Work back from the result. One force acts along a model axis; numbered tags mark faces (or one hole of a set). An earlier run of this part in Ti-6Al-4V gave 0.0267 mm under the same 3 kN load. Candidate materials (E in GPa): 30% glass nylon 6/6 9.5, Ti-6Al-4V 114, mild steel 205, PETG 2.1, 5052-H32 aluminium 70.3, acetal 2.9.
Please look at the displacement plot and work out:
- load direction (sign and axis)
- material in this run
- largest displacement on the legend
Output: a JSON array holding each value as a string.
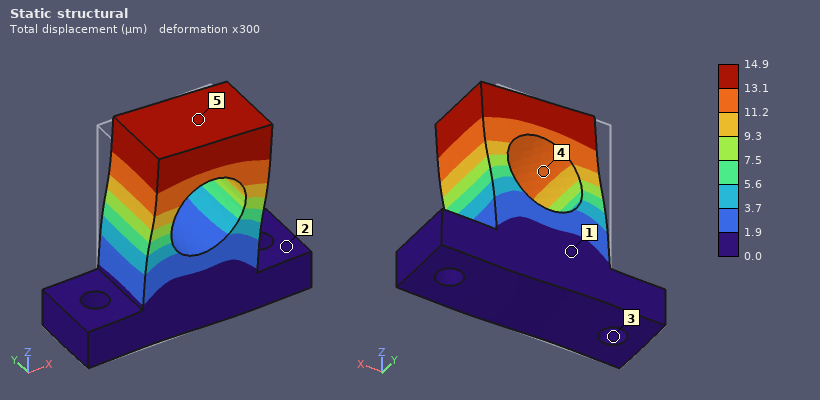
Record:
["+X", "mild steel", "14.9 µm"]
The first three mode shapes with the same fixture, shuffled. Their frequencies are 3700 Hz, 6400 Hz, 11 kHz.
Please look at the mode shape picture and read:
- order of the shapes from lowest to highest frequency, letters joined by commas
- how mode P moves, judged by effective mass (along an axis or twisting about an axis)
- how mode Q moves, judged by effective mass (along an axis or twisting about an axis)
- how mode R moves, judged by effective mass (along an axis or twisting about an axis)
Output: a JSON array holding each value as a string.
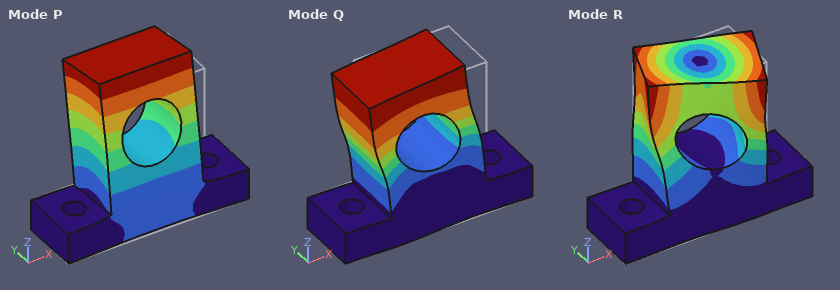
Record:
["P, Q, R", "along Y", "along X", "twisting about Z"]
